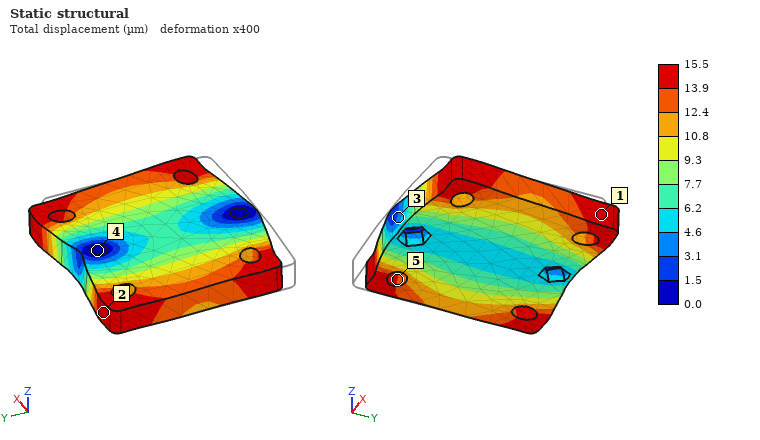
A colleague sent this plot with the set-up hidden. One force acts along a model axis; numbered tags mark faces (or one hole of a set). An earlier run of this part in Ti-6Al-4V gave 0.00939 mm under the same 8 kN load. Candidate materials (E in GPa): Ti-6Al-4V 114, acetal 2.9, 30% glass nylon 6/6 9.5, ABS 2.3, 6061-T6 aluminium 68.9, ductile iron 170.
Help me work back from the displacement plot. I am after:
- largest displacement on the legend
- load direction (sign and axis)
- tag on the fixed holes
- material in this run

15.5 µm
+Y
4
6061-T6 aluminium
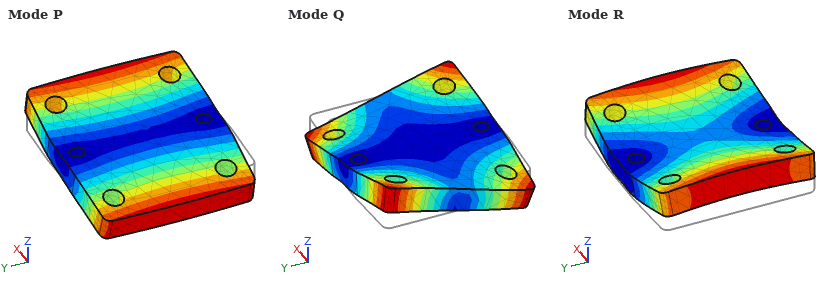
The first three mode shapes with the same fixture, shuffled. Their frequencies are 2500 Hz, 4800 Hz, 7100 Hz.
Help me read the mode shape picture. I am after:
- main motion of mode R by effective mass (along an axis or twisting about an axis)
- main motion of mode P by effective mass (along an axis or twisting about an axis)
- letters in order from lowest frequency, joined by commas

along Z
twisting about Y
P, R, Q
